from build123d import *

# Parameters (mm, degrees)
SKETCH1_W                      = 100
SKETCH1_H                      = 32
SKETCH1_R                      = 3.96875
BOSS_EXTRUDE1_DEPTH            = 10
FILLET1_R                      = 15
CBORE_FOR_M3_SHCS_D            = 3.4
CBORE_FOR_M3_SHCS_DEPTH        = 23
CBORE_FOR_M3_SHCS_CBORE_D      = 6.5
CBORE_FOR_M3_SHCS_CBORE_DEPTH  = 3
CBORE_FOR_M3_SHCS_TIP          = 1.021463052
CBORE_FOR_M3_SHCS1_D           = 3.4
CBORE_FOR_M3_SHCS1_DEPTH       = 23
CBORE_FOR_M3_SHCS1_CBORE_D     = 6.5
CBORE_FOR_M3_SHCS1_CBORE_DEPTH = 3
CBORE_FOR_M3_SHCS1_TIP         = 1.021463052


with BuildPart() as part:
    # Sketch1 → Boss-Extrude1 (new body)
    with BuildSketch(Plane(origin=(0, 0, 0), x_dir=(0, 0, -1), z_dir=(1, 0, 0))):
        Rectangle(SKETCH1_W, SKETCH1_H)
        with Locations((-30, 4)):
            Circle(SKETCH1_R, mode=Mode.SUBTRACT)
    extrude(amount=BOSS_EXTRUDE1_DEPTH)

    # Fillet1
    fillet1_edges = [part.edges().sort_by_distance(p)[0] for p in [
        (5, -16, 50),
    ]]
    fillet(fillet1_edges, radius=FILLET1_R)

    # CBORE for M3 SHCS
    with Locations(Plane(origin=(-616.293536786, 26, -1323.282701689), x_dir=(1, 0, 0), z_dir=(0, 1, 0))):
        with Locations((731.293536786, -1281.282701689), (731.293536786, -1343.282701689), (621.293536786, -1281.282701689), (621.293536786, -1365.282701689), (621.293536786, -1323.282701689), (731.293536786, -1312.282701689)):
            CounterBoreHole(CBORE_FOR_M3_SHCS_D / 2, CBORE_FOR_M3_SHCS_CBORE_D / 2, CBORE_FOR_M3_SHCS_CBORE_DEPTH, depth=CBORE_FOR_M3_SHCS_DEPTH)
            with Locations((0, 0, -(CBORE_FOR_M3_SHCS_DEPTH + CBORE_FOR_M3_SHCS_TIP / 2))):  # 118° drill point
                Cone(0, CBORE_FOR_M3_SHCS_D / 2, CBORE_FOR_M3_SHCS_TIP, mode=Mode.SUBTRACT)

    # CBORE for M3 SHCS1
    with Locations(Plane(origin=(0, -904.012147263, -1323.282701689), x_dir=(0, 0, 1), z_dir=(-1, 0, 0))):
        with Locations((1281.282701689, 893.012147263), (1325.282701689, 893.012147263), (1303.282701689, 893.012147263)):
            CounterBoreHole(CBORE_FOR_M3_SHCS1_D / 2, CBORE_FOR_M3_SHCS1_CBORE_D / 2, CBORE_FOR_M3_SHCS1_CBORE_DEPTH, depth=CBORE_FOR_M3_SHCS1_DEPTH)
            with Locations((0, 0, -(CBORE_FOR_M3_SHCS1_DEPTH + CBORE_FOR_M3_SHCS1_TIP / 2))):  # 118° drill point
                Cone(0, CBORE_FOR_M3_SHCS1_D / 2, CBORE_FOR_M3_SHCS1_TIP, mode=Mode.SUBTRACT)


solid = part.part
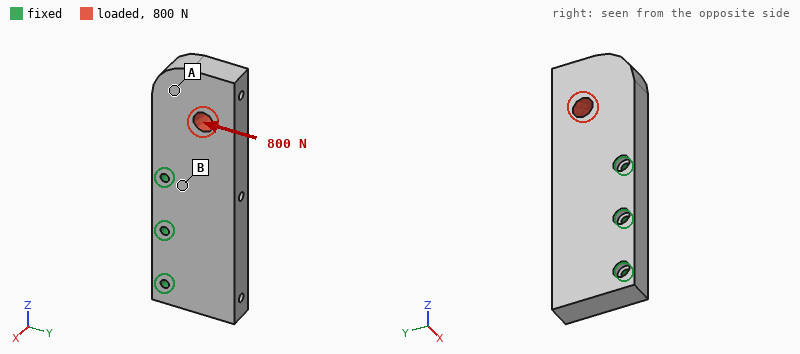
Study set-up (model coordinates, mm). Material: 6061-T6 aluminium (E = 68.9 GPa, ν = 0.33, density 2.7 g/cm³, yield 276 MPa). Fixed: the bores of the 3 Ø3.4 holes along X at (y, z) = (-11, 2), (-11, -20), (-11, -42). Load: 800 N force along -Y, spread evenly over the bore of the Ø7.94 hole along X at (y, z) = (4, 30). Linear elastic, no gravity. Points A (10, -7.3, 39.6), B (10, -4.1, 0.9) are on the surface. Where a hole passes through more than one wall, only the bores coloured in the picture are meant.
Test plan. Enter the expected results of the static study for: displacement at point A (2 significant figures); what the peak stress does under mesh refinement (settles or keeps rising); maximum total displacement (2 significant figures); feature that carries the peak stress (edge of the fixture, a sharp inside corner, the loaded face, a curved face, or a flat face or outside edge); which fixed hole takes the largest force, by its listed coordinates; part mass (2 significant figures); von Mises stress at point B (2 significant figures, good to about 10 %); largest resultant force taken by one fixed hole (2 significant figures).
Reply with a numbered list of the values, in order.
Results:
1. 17 µm
2. keeps rising
3. 24 µm
4. edge of the fixture
5. (-11, 2)
6. 81 g
7. 8.7 MPa
8. 1.4 kN
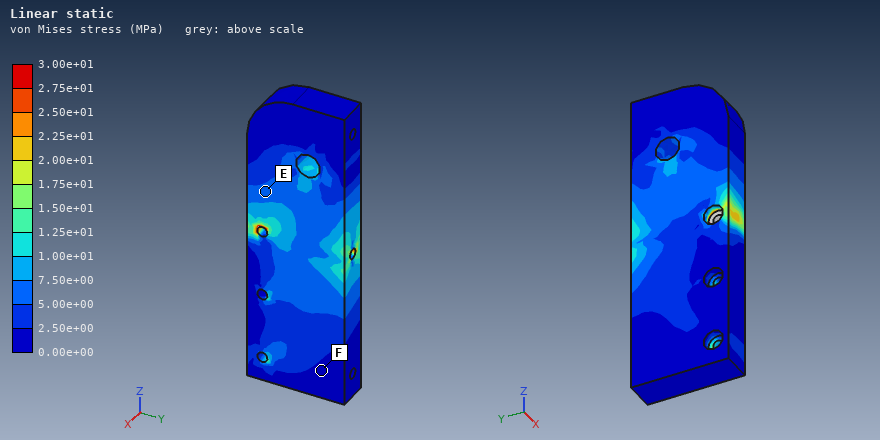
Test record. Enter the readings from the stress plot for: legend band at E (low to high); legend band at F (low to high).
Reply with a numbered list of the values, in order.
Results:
1. 5.00e+00 to 7.50e+00 MPa
2. 0.00e+00 to 2.50e+00 MPa
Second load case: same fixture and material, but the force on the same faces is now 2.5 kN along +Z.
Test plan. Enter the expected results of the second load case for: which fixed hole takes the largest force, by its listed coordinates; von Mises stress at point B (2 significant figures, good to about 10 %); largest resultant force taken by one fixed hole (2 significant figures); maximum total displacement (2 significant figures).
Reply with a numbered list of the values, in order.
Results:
1. (-11, 2)
2. 12 MPa
3. 1.4 kN
4. 25 µm
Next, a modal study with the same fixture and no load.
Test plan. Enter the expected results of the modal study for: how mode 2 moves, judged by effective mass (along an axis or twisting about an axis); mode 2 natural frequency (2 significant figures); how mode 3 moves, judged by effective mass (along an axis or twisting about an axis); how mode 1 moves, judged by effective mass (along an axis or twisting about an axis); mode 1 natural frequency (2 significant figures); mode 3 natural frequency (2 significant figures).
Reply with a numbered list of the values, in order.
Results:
1. along X
2. 5800 Hz
3. along Y
4. along X
5. 2600 Hz
6. 6300 Hz
